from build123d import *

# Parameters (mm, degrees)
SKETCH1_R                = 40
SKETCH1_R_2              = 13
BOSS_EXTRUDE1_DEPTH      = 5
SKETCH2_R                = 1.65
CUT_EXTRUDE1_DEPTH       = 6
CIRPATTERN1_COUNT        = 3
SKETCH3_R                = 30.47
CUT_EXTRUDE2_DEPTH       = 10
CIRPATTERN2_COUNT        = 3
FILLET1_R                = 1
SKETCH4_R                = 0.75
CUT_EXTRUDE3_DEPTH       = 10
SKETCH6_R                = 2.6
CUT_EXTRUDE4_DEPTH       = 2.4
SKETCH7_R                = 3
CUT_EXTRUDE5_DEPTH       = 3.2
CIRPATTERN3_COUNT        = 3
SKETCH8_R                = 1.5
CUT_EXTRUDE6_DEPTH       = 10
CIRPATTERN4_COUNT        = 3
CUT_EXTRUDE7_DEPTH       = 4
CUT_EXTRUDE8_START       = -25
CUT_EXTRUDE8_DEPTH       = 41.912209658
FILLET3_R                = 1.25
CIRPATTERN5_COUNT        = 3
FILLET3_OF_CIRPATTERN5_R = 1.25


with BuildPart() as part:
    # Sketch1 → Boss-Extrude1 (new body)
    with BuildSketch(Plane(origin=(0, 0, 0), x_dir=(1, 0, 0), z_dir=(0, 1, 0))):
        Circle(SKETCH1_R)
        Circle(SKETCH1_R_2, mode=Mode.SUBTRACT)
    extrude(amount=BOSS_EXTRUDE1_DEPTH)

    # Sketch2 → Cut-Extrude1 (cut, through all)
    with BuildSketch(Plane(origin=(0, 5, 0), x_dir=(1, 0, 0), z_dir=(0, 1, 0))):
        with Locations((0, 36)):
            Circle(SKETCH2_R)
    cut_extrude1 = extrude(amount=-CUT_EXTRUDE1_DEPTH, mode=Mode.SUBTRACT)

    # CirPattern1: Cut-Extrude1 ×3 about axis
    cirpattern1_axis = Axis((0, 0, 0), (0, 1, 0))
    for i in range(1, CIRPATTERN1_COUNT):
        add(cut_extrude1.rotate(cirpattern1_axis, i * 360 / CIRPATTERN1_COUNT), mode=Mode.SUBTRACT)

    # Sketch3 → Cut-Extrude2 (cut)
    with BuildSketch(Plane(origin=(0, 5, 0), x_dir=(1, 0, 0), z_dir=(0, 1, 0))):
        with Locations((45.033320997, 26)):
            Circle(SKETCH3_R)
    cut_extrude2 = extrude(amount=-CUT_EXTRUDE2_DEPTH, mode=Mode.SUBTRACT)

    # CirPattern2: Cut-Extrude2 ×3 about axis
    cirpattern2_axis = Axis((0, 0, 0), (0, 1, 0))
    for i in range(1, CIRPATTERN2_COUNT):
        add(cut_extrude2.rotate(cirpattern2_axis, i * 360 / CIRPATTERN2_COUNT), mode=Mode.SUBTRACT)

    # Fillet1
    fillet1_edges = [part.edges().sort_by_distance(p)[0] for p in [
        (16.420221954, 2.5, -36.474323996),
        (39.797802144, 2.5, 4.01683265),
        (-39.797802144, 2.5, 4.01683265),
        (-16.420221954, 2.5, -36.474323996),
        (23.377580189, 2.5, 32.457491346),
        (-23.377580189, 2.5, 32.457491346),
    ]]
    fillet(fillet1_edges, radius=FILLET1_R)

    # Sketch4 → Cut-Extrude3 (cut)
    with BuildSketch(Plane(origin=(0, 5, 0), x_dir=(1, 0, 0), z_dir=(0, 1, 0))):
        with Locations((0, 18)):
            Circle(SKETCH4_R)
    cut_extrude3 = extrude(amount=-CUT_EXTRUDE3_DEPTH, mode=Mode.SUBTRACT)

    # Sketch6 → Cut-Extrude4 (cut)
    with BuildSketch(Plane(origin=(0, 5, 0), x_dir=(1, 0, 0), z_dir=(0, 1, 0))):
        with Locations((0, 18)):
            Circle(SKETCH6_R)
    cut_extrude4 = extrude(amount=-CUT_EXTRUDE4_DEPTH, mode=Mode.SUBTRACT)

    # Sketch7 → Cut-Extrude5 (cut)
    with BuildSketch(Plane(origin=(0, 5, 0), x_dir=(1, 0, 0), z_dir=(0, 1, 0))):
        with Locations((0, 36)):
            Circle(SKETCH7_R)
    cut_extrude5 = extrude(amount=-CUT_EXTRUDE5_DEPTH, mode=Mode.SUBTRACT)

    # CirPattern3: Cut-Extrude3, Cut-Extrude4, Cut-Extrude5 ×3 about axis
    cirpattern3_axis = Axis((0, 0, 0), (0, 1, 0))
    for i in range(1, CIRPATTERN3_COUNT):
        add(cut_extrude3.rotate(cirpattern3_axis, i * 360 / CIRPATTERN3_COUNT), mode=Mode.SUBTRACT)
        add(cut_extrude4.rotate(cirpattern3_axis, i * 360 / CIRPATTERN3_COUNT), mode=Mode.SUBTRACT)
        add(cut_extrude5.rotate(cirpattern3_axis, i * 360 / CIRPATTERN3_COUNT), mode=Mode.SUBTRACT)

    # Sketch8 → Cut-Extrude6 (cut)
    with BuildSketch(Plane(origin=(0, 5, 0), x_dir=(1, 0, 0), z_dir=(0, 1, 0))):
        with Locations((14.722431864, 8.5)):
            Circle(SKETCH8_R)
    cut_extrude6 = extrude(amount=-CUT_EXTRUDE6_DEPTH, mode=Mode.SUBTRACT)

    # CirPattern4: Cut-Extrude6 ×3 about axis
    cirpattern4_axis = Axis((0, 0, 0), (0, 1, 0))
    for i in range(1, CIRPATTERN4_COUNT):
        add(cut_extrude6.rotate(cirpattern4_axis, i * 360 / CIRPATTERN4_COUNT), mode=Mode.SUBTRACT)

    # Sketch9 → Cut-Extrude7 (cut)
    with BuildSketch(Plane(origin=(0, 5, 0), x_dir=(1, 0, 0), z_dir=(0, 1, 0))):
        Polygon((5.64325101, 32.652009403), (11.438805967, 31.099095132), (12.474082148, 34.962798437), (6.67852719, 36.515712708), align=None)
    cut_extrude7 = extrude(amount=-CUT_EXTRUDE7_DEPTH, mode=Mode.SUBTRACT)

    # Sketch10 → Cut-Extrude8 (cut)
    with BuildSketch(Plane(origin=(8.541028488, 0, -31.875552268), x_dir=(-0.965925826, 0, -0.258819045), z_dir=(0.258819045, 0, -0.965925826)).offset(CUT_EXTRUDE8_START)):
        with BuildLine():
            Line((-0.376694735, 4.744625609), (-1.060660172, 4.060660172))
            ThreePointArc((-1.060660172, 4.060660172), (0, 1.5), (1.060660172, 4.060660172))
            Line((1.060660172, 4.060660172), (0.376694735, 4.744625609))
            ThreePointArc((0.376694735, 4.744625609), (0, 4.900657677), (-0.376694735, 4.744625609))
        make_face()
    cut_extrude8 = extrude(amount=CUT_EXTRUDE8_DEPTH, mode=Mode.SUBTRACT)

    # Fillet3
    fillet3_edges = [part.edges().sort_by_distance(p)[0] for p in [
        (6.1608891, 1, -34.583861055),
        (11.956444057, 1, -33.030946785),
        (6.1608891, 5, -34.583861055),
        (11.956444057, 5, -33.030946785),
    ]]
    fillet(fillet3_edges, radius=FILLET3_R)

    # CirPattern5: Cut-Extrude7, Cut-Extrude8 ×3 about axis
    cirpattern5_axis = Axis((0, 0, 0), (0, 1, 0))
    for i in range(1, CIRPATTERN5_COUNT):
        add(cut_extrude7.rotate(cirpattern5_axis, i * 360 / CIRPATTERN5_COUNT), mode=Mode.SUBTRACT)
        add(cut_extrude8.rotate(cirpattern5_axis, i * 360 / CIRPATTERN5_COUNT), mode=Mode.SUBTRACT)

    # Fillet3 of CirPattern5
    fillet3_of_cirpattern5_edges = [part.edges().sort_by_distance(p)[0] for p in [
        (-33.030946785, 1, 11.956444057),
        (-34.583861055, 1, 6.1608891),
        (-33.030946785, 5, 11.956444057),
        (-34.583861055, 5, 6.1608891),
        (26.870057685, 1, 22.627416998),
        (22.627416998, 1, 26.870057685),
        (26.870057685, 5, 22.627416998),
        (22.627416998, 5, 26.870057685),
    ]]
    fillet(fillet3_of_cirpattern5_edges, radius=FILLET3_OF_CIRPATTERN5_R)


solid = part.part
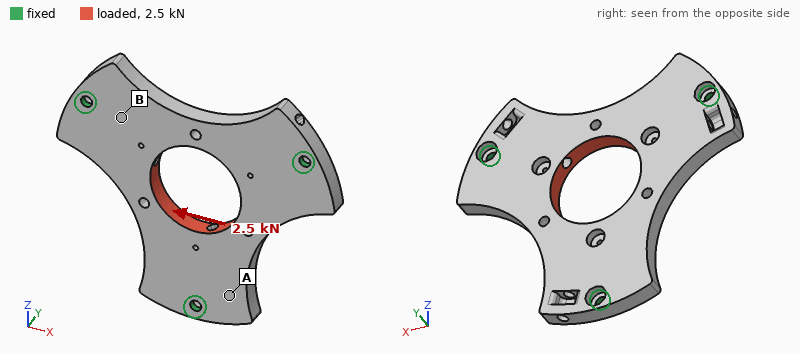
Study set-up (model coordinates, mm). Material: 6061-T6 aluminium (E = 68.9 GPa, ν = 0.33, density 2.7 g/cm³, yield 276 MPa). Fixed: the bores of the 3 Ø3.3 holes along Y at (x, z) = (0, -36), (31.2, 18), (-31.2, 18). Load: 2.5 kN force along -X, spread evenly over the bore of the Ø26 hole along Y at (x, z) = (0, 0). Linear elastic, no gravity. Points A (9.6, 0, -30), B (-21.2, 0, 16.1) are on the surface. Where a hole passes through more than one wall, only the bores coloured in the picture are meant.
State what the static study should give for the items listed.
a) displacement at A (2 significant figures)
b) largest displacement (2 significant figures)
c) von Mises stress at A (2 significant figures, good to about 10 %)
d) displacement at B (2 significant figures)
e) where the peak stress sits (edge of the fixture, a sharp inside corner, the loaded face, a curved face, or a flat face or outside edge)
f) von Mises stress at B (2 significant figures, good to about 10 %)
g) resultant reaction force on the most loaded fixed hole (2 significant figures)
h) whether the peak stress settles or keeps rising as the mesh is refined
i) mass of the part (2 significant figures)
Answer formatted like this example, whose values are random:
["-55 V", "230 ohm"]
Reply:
["12 µm", "30 µm", "10 MPa", "7.4 µm", "a sharp inside corner", "22 MPa", "1.1 kN", "keeps rising", "33 g"]
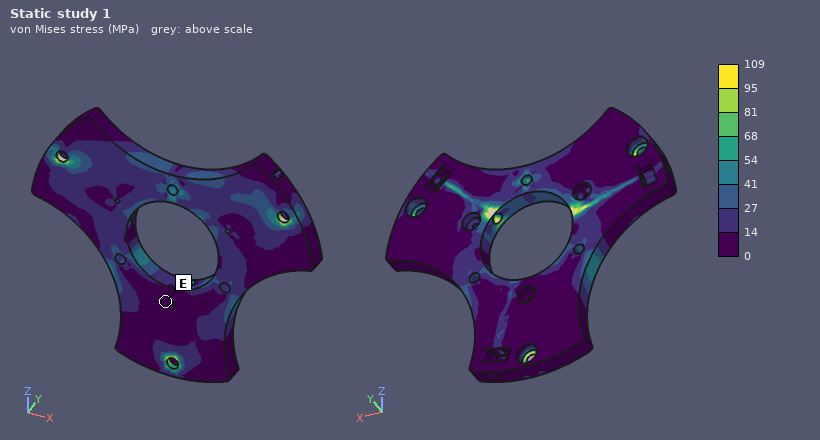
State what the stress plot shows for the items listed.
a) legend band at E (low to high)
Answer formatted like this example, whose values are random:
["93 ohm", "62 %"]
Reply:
["0 to 14 MPa"]
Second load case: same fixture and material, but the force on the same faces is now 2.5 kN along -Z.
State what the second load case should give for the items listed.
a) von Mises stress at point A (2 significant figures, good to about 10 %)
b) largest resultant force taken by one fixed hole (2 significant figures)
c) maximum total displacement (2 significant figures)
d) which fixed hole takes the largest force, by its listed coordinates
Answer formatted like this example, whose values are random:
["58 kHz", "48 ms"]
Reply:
["22 MPa", "1.2 kN", "33 µm", "(0, -36)"]
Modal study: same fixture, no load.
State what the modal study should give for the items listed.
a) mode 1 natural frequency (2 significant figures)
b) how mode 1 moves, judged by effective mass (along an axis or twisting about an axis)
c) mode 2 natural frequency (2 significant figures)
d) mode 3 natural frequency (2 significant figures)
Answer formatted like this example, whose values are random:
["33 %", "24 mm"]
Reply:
["4300 Hz", "along Y", "5500 Hz", "5500 Hz"]
